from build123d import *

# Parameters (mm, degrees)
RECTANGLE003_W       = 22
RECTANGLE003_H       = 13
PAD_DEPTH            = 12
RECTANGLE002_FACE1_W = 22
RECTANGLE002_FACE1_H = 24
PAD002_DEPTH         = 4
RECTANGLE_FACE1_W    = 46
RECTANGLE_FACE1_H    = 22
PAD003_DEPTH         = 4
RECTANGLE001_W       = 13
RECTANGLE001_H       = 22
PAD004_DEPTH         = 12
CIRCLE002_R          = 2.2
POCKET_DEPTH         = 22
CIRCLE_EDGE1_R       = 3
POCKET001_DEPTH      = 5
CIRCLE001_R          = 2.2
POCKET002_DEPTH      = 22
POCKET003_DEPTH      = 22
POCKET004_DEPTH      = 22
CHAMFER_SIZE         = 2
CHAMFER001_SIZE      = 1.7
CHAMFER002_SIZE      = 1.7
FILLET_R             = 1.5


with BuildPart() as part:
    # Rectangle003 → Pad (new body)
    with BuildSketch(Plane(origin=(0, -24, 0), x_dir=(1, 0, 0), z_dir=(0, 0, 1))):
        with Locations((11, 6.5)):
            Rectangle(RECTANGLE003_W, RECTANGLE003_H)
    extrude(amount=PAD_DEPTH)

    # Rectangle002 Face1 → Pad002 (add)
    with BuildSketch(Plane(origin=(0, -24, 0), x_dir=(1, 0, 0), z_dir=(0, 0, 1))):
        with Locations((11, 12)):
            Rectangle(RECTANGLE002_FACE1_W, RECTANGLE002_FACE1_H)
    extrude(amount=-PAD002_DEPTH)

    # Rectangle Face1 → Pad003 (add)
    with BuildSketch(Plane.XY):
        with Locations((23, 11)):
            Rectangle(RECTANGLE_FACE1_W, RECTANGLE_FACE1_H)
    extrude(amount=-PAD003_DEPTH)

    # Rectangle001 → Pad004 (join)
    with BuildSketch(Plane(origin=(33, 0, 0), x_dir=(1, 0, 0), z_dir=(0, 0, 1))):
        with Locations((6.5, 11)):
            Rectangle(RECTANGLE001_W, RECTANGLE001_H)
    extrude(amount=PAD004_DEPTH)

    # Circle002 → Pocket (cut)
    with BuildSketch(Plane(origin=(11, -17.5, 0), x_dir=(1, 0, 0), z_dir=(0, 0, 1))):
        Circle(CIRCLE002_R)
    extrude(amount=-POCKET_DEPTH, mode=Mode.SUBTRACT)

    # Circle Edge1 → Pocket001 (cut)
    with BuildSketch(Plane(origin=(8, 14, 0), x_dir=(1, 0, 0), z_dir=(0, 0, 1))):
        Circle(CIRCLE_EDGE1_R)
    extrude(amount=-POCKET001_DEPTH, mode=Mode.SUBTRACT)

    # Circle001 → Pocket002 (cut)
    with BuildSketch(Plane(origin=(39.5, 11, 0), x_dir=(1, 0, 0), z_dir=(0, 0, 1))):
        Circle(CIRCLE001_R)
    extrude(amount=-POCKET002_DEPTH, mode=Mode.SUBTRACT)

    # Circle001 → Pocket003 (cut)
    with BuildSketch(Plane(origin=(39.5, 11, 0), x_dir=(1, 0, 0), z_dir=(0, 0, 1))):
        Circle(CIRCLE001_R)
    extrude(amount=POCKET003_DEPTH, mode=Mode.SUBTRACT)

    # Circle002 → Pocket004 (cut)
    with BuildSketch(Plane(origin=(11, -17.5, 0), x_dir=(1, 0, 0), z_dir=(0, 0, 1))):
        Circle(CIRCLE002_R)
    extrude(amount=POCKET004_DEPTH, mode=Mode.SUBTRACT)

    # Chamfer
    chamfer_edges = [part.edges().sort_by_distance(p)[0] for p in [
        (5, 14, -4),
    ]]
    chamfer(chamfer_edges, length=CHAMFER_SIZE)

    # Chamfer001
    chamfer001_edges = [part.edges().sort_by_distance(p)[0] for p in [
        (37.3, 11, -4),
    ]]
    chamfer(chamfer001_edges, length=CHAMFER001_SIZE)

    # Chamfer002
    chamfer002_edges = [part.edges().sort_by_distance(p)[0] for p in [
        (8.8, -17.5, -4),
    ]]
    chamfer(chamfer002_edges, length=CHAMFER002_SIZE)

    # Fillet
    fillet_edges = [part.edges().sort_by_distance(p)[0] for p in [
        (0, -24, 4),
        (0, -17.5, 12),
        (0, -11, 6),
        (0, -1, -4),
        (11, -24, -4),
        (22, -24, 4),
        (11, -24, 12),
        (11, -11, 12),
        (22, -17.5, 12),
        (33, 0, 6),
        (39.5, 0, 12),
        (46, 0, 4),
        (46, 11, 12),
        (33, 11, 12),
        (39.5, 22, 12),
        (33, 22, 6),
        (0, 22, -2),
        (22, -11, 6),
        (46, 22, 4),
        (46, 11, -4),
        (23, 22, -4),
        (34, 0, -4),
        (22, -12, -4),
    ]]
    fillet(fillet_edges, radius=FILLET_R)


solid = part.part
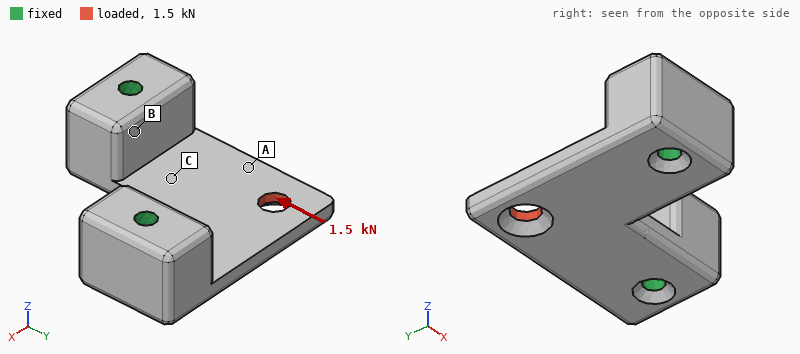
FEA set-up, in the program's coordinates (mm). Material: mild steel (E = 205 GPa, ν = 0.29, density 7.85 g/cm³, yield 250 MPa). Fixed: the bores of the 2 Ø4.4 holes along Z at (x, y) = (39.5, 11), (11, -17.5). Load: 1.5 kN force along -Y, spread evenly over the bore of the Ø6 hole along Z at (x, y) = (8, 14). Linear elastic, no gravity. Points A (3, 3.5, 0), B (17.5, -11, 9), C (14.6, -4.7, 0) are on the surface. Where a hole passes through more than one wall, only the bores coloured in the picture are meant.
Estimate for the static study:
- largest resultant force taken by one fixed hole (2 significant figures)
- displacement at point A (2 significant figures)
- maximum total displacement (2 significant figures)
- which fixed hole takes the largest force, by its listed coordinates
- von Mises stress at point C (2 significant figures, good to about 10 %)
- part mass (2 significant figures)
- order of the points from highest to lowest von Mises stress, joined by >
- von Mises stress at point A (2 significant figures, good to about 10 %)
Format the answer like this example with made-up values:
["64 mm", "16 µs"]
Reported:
["1.4 kN", "3.1 µm", "14 µm", "(11, -17.5)", "23 MPa", "95 g", "A > C > B", "39 MPa"]
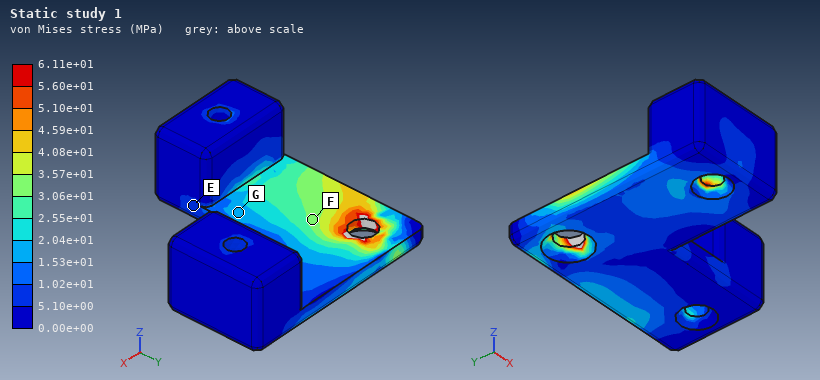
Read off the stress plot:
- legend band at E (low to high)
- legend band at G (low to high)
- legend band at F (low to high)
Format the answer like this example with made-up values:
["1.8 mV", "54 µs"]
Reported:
["5.10e+00 to 1.02e+01 MPa", "1.53e+01 to 2.04e+01 MPa", "3.06e+01 to 3.57e+01 MPa"]
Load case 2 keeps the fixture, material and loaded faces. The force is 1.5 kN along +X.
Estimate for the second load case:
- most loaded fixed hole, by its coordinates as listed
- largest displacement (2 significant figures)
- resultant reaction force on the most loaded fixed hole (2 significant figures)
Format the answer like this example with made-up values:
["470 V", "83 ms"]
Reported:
["(39.5, 11)", "14 µm", "1.4 kN"]
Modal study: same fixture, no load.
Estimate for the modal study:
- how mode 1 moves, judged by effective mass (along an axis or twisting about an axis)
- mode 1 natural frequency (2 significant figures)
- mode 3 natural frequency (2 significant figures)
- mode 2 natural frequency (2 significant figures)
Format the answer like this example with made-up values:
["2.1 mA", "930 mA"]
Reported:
["along Z", "5300 Hz", "18 kHz", "16 kHz"]
